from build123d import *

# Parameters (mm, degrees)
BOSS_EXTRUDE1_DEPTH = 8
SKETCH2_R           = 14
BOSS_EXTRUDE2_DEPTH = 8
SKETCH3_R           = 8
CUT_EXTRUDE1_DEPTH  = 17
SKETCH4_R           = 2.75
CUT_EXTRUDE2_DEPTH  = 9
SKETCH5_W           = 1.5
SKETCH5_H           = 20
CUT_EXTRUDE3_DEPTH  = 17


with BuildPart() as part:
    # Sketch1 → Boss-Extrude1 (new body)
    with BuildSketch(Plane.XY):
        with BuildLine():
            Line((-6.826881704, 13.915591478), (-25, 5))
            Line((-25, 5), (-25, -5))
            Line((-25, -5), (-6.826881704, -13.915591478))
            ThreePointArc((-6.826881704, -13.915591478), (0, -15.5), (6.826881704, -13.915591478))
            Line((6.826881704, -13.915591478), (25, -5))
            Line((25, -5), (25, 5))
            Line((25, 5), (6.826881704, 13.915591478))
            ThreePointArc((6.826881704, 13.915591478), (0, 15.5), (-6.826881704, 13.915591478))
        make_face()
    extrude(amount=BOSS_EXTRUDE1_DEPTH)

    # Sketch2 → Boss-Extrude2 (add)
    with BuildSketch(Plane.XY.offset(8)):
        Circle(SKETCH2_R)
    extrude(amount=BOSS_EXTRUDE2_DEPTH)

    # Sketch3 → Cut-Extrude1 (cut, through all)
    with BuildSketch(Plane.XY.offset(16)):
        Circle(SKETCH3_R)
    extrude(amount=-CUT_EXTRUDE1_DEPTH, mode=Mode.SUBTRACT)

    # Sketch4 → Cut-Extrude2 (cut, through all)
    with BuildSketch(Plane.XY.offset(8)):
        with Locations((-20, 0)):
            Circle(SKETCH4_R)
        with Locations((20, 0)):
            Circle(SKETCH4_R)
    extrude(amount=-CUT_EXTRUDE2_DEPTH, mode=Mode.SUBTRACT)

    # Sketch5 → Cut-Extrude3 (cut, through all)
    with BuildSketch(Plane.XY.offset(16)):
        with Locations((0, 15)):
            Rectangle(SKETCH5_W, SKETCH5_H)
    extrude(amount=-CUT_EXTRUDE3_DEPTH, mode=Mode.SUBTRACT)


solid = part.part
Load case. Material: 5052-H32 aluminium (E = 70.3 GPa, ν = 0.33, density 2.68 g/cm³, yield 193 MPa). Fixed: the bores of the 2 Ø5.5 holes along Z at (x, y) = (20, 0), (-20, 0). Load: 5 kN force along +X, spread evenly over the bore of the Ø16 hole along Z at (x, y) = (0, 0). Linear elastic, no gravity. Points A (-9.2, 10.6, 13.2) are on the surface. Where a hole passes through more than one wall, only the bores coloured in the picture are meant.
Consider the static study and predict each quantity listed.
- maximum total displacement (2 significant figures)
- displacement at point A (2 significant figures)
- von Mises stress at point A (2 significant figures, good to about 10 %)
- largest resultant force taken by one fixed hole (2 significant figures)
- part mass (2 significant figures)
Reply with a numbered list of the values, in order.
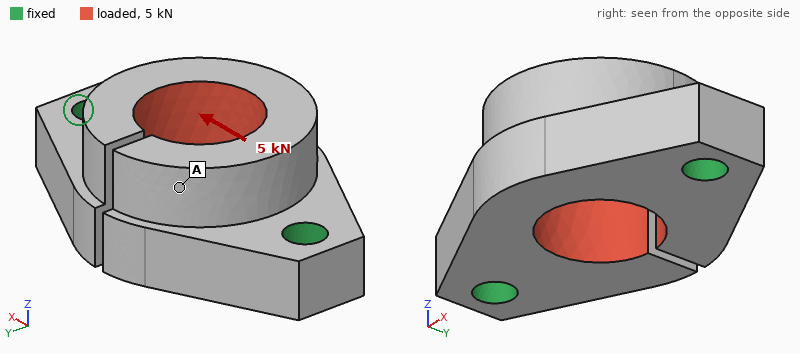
1. 25 µm
2. 16 µm
3. 8.9 MPa
4. 2.5 kN
5. 27 g
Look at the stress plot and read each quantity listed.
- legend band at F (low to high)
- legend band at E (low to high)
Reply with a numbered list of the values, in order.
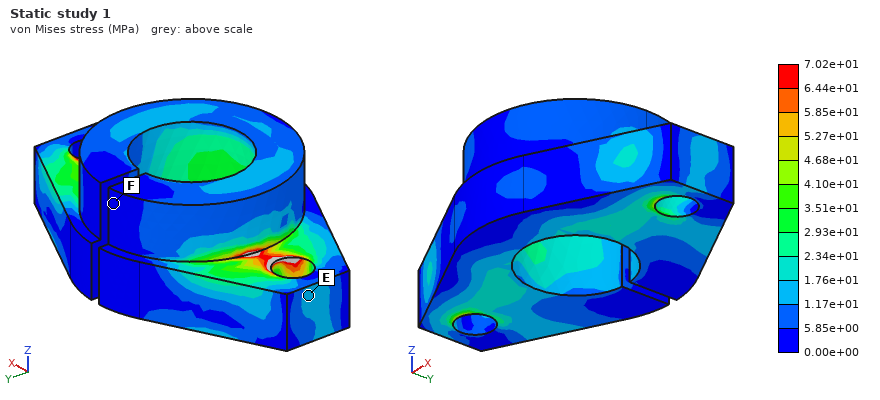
1. 0.00e+00 to 5.85e+00 MPa
2. 1.17e+01 to 1.76e+01 MPa
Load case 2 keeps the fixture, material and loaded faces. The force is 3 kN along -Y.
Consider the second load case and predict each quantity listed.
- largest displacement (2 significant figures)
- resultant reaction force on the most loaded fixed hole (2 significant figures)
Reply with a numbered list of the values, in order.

1. 33 µm
2. 1.8 kN
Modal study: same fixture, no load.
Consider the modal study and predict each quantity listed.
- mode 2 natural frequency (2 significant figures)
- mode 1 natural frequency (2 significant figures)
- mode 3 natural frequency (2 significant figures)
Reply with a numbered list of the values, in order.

1. 13 kHz
2. 13 kHz
3. 14 kHz
